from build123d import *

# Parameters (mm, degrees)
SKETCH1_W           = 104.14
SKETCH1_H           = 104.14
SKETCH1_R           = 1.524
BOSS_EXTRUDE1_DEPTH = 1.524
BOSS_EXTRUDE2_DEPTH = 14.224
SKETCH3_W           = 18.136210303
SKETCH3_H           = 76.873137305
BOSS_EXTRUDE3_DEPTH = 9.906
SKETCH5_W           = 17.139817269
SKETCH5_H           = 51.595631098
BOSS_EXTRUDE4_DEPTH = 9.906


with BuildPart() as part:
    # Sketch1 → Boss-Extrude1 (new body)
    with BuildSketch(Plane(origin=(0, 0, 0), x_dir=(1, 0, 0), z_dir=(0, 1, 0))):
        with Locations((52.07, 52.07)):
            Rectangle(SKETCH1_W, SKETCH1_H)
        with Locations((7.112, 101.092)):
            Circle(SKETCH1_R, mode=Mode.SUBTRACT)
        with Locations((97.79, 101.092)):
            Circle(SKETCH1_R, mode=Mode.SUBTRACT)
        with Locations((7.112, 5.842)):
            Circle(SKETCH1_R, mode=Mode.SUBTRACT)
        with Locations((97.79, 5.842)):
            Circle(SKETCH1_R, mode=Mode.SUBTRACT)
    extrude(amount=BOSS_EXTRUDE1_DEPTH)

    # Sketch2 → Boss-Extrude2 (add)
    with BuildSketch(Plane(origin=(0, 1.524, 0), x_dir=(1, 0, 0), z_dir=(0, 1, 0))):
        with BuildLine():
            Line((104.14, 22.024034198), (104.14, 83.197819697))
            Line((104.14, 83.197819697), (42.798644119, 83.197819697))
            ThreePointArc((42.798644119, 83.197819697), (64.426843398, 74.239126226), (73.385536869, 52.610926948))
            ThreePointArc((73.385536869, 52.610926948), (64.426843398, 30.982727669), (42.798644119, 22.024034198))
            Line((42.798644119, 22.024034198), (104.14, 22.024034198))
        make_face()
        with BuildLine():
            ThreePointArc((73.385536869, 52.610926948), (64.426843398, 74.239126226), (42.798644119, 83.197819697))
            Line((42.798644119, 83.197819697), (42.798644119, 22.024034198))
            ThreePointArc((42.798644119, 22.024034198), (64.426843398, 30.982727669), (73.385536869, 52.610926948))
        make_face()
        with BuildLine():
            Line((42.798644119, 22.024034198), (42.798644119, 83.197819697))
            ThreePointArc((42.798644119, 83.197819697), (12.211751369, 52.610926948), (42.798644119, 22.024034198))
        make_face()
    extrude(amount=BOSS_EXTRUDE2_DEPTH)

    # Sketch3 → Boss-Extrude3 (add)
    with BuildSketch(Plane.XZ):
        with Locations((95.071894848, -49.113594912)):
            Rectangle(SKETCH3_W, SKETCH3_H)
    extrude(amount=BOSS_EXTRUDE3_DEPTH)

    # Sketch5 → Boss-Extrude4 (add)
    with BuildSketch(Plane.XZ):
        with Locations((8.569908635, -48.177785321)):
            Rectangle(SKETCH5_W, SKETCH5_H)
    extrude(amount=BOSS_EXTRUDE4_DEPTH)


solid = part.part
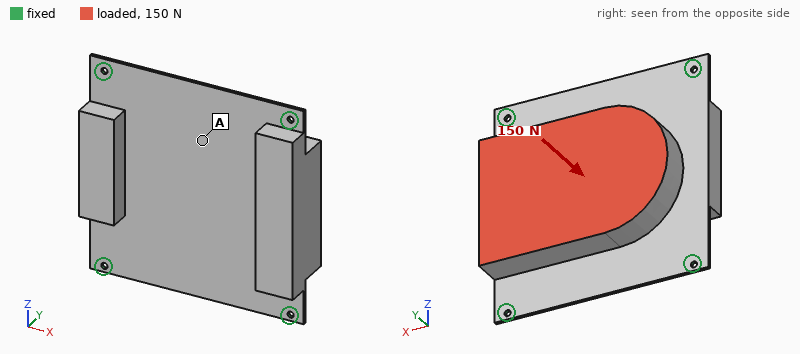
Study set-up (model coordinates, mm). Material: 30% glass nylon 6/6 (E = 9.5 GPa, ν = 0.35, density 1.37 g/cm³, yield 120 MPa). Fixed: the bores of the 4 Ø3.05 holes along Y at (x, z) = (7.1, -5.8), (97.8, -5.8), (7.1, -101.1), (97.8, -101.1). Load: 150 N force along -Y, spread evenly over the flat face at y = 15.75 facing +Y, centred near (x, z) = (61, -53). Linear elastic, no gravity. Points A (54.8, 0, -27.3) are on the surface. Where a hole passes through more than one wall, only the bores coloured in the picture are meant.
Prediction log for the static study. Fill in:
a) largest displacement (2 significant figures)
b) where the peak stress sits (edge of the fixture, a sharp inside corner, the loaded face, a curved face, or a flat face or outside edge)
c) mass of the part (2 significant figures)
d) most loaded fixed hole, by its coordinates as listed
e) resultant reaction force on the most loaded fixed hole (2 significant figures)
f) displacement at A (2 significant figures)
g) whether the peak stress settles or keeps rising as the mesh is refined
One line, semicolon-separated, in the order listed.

0.41 mm; edge of the fixture; 160 g; (97.8, -101.1); 54 N; 0.18 mm; keeps rising
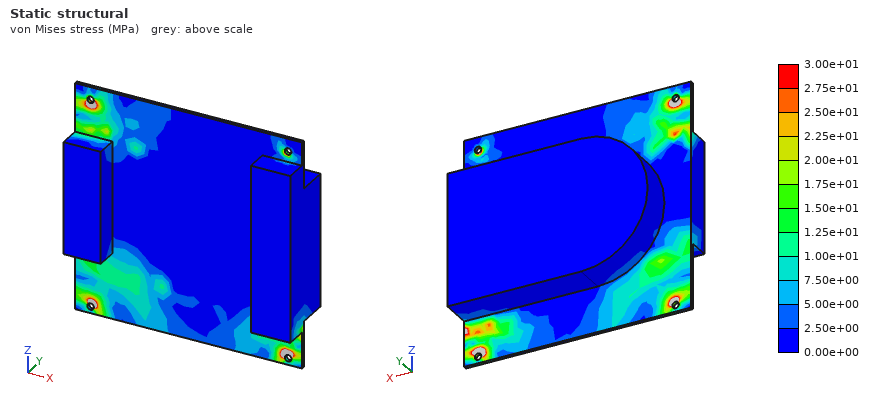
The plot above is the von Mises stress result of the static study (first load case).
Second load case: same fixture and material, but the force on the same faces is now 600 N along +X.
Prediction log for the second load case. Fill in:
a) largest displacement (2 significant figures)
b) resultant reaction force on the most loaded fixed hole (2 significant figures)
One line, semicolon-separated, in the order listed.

0.53 mm; 190 N
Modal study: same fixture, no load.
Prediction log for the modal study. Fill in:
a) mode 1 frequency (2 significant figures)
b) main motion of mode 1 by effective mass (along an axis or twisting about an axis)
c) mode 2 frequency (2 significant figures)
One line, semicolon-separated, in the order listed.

310 Hz; along Y; 580 Hz
